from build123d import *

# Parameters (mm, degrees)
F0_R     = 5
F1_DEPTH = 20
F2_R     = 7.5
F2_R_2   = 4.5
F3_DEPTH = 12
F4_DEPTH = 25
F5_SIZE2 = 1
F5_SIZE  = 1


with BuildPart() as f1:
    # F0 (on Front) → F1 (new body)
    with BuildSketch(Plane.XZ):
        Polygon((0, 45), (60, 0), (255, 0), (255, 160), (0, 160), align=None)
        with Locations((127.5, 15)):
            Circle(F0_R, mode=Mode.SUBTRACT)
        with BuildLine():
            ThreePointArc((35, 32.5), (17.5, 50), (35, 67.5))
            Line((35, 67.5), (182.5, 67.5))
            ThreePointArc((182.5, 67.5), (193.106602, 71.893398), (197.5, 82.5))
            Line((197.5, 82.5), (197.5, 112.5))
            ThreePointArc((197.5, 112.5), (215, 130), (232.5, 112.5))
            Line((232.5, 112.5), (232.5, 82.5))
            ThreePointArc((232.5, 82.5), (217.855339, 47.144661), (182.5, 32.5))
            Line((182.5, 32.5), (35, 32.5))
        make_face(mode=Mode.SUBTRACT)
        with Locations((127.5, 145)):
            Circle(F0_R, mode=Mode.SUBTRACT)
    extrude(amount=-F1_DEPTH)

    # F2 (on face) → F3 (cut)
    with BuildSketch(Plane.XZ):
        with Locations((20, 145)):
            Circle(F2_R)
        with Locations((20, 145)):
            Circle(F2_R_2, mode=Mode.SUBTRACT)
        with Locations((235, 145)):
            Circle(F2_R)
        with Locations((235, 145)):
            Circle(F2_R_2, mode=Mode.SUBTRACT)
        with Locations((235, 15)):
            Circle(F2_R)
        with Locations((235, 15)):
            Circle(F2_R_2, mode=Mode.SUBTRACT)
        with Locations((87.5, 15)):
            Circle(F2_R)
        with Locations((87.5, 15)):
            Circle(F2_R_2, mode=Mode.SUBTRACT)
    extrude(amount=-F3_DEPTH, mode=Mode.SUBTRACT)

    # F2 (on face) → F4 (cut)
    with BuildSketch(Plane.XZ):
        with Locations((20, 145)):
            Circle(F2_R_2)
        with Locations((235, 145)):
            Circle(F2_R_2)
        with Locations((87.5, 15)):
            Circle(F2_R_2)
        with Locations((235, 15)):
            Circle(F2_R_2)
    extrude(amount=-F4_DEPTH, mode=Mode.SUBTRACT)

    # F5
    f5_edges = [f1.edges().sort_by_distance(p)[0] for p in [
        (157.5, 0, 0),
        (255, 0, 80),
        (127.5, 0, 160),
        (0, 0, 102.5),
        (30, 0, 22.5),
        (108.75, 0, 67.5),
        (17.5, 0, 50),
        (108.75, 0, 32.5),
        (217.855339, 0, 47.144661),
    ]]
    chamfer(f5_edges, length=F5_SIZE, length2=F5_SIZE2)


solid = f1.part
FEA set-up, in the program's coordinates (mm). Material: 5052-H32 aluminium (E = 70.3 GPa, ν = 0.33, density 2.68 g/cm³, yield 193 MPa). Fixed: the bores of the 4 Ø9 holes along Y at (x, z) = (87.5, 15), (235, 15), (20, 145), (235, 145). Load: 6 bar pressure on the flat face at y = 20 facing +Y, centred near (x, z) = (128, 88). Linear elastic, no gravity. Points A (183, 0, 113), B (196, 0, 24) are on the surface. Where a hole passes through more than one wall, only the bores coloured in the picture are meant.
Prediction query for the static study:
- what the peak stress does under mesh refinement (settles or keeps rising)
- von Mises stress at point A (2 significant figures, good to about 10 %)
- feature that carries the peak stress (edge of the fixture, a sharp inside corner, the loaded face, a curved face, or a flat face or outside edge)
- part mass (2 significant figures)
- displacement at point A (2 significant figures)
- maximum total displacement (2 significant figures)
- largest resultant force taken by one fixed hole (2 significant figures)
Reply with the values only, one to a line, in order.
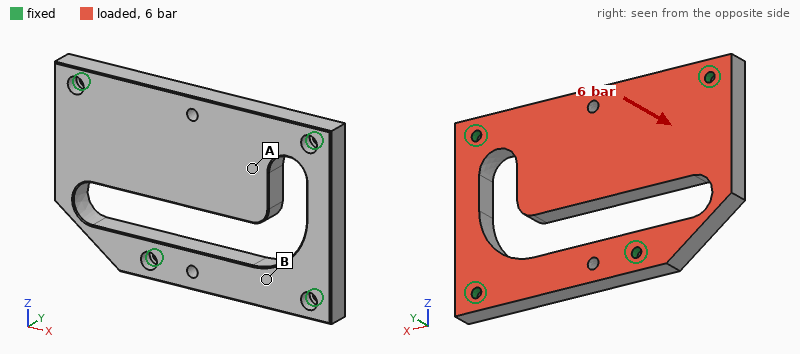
keeps rising
30 MPa
edge of the fixture
1.6 kg
0.26 mm
0.48 mm
7.5 kN
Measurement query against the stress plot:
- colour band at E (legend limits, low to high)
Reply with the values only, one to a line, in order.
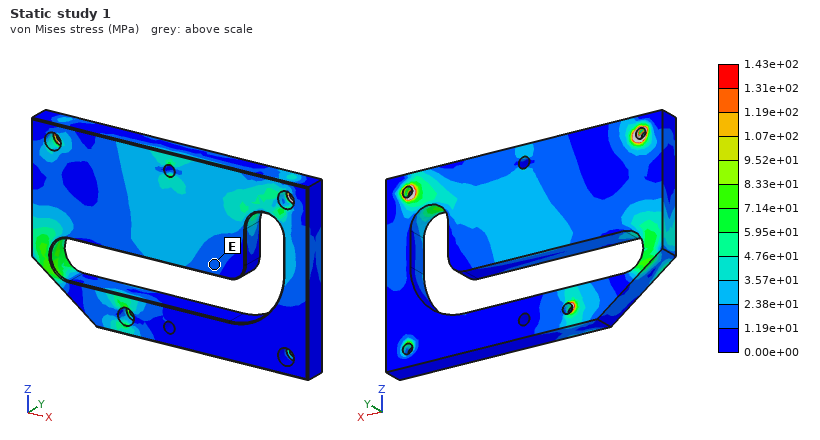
1.19e+01 to 2.38e+01 MPa
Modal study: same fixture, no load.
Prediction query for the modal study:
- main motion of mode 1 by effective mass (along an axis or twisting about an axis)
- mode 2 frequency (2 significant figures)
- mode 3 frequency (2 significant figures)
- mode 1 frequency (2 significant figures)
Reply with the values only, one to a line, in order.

along Y
1900 Hz
2600 Hz
1000 Hz
